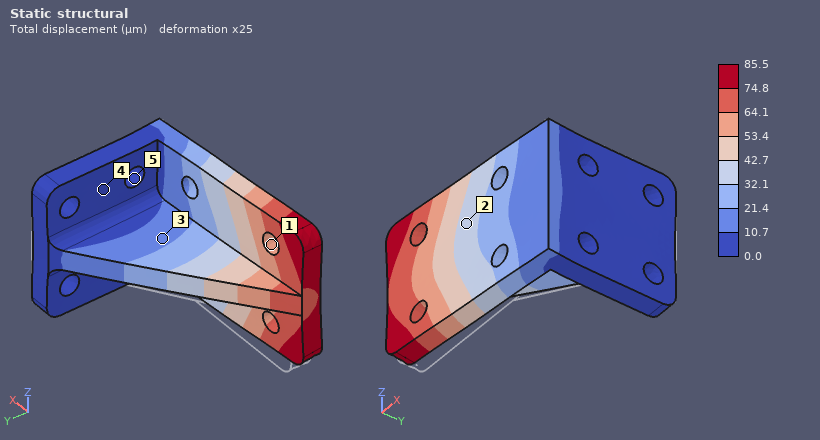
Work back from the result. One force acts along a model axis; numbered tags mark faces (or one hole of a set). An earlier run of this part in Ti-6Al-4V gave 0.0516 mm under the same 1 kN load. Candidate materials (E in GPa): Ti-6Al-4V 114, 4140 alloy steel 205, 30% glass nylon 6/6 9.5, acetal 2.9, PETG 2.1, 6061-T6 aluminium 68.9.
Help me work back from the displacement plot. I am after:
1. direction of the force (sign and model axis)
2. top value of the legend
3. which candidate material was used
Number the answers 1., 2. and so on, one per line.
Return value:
1. -Y
2. 85.5 µm
3. 6061-T6 aluminium
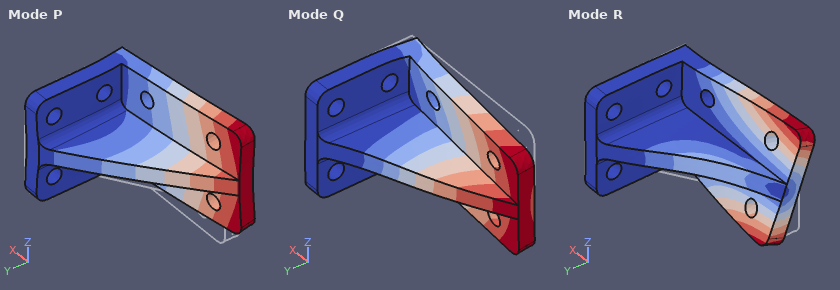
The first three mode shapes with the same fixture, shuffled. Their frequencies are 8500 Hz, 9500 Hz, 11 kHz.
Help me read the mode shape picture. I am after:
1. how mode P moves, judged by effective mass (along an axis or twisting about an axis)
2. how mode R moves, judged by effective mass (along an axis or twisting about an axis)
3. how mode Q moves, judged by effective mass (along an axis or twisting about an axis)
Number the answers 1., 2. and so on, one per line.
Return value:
1. along Y
2. twisting about X
3. along Z
